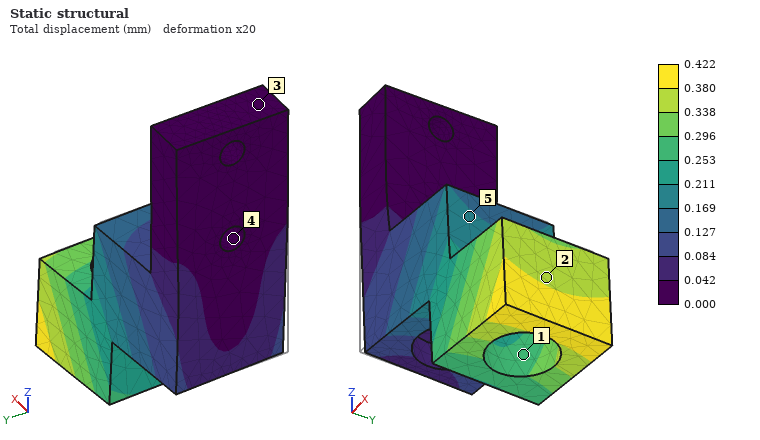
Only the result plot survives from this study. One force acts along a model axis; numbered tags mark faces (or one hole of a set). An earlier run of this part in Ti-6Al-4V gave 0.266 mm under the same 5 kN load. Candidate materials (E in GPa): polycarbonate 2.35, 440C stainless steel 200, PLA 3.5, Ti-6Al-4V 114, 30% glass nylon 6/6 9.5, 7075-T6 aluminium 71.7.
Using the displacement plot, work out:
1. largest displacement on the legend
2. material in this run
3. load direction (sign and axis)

0.422 mm
7075-T6 aluminium
+Y
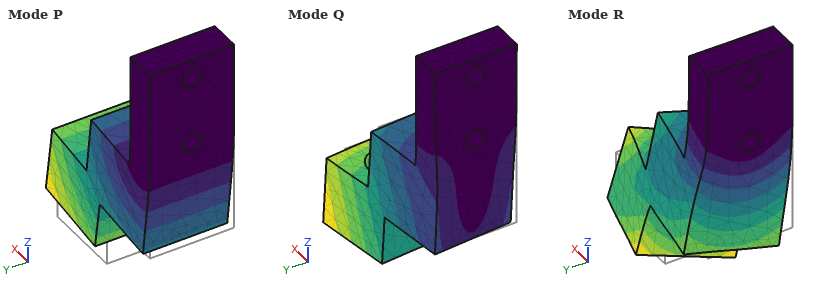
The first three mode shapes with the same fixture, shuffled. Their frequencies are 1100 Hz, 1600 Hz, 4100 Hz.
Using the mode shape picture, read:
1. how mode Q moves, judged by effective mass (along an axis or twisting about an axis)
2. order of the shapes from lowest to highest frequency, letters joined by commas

along Y
P, Q, R
